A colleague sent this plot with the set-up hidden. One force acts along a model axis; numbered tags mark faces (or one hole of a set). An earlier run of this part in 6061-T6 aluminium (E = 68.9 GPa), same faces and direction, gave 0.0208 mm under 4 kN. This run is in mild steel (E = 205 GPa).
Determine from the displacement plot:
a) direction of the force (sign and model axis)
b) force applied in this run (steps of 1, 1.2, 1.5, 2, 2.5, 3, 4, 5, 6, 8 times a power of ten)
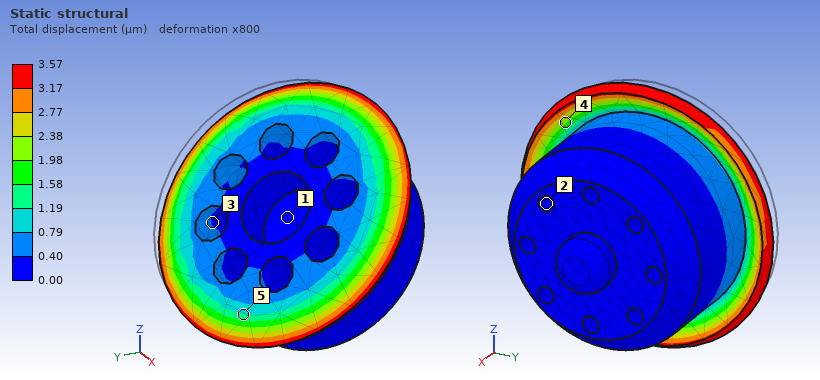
+X
2 kN
